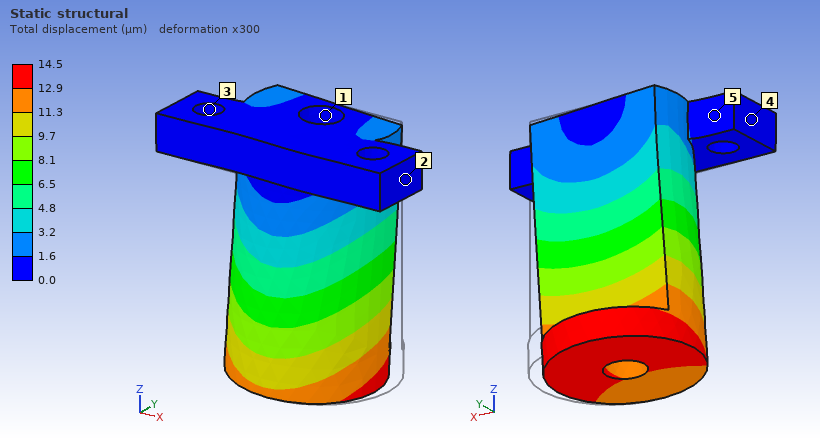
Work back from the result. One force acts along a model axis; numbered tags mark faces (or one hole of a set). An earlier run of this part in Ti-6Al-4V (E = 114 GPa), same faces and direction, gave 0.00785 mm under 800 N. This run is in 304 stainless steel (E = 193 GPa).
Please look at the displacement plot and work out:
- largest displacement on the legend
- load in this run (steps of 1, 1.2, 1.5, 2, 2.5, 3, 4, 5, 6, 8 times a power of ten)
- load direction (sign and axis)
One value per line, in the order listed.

14.5 µm
2.5 kN
-X
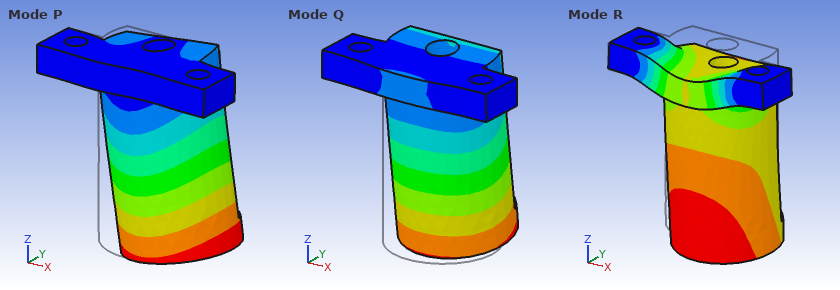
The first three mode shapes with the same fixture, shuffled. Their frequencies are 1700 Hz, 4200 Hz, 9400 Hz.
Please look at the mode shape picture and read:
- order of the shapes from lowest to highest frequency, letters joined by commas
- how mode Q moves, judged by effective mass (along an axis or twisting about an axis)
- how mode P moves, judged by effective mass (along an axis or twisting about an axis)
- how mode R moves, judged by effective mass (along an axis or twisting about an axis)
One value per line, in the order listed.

Q, P, R
along Y
along X
along Z
